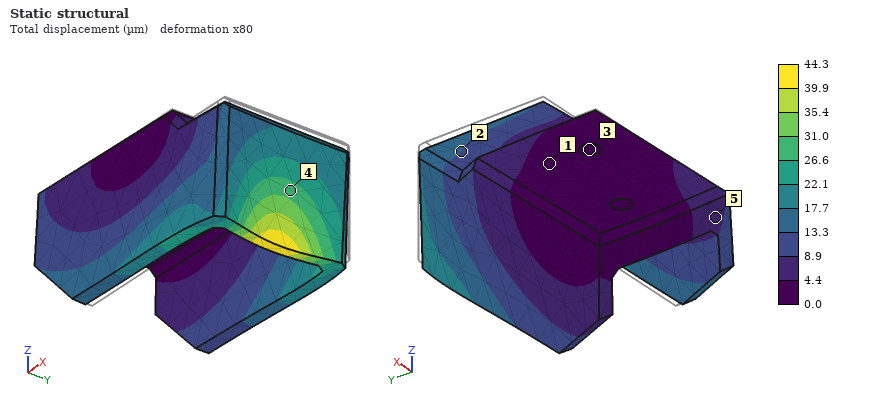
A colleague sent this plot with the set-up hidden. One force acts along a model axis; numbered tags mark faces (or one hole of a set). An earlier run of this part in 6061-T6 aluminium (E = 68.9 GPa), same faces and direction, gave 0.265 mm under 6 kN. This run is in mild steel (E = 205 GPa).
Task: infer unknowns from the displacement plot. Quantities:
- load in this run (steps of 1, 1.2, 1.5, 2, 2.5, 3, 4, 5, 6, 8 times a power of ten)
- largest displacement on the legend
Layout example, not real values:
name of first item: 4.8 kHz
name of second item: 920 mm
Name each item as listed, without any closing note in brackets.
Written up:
load in this run: 3 kN
largest displacement on the legend: 44.3 µm
